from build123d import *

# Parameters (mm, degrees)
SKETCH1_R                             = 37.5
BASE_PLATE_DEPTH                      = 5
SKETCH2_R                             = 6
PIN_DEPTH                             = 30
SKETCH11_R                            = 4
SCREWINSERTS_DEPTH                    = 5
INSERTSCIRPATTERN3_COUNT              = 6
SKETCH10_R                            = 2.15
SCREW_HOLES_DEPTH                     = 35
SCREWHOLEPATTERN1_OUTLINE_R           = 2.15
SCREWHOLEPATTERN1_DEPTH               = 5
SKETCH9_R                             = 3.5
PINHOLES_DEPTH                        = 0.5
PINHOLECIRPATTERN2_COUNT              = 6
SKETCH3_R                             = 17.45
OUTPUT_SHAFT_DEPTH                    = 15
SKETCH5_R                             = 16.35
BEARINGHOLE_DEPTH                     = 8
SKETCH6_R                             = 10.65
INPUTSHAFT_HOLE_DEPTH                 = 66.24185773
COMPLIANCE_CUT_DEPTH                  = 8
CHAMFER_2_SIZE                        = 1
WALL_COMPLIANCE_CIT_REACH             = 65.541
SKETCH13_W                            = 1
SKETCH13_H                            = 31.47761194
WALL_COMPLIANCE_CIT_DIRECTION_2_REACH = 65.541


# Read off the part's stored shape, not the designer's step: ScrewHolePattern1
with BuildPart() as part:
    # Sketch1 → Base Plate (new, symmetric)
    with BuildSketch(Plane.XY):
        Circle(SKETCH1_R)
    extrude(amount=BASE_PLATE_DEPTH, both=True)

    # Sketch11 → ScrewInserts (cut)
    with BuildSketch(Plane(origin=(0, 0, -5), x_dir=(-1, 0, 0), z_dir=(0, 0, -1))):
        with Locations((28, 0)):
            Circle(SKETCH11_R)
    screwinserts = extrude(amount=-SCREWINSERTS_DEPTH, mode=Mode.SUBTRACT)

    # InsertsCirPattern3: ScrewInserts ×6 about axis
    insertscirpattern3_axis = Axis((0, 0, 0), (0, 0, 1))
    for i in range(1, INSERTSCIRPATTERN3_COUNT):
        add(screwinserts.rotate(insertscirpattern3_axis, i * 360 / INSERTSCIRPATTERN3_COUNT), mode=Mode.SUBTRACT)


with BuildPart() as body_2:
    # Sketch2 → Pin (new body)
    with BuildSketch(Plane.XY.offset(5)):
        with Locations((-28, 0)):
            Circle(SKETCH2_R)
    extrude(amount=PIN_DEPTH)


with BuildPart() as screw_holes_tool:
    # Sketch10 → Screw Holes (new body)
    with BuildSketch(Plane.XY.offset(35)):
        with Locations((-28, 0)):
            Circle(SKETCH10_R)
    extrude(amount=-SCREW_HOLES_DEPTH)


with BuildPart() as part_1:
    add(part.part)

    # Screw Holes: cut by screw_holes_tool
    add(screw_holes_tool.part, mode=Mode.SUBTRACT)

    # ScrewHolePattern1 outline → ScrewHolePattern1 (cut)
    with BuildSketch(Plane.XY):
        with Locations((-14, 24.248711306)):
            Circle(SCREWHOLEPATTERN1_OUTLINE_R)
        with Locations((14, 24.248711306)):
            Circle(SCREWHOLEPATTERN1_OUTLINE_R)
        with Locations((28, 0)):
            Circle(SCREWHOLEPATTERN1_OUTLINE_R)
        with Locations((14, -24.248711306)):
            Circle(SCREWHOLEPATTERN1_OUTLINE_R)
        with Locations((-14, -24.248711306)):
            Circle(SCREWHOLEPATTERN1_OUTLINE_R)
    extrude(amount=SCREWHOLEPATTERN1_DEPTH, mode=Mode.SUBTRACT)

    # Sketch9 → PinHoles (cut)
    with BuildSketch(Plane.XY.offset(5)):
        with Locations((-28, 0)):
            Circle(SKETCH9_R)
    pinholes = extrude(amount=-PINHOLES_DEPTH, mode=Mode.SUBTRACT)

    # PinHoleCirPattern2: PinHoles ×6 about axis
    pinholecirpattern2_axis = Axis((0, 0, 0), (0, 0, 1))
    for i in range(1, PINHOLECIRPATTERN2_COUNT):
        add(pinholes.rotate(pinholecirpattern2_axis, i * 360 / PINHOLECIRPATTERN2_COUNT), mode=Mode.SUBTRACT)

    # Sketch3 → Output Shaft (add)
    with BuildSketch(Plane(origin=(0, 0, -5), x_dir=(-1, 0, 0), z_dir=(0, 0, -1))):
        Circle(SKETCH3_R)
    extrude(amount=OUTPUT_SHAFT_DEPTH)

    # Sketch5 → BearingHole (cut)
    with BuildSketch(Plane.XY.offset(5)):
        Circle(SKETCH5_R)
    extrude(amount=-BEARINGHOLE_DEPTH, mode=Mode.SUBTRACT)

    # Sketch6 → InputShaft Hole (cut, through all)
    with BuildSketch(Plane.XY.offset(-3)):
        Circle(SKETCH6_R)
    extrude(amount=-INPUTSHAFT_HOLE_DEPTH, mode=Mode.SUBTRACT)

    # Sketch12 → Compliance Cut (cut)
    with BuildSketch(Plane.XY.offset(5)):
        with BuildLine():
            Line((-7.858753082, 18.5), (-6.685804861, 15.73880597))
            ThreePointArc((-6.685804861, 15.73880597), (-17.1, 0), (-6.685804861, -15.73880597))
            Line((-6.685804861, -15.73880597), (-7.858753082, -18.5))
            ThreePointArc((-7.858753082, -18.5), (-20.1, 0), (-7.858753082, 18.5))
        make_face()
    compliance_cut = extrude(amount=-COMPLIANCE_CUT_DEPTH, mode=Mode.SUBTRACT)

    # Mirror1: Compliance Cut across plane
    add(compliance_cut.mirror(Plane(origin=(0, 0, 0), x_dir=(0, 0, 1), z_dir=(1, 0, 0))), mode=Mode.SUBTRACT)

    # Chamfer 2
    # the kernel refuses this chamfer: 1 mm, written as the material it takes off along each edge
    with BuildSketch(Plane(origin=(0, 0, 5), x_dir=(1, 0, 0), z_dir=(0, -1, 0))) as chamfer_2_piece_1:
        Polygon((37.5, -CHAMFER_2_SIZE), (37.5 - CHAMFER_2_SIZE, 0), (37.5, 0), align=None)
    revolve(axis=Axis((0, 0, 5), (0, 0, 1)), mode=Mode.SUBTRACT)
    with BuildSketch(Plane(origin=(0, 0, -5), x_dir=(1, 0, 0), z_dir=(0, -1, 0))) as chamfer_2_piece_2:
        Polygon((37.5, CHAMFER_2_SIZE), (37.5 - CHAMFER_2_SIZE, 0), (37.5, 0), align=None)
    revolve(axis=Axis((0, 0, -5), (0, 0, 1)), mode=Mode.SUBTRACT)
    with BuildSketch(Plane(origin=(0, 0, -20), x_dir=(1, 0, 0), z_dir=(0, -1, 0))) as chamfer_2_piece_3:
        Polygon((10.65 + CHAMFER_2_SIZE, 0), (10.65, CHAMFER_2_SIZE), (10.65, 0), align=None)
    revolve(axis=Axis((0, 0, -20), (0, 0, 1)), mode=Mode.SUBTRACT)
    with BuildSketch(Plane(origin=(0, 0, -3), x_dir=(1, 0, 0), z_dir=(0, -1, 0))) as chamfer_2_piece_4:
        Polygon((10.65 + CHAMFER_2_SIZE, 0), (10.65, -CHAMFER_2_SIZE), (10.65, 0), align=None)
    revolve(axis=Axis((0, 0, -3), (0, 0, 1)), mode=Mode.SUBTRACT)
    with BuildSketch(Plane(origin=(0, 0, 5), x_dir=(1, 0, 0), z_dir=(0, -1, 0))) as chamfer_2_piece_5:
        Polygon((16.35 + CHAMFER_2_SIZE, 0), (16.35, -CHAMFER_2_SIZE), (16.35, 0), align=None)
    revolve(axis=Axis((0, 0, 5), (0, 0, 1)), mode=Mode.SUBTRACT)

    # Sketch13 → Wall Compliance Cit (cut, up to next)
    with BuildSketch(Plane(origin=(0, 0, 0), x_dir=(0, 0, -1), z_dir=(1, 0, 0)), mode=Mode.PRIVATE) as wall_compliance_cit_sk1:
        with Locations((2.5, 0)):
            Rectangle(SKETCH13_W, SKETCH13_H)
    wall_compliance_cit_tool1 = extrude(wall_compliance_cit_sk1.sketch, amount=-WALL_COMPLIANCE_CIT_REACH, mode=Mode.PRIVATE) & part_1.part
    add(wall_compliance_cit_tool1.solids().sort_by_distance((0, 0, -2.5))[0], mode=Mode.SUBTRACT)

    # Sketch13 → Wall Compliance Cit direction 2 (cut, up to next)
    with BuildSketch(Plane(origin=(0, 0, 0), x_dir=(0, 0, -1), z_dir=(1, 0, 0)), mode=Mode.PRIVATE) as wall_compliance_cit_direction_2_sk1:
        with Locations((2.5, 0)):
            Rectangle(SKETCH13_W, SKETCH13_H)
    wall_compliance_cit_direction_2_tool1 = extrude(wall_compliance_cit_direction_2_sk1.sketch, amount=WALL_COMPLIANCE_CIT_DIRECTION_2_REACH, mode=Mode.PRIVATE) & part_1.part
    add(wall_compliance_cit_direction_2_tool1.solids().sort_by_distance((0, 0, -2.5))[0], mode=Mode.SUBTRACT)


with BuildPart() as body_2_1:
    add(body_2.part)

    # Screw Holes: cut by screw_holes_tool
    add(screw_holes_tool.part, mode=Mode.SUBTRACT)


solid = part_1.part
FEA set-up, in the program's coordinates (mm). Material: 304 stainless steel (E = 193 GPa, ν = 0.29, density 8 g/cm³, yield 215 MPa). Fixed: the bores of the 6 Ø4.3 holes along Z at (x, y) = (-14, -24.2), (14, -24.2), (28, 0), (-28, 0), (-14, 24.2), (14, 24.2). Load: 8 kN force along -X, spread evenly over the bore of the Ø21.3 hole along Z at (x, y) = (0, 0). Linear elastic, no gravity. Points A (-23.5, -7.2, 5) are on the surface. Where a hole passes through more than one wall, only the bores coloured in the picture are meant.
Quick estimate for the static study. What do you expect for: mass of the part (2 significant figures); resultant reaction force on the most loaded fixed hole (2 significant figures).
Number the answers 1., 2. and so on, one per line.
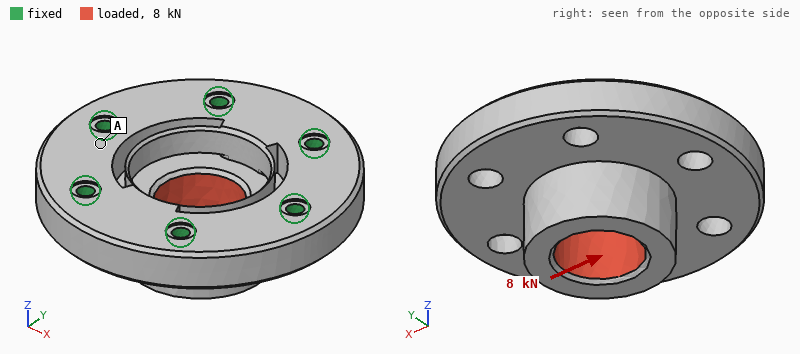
1. 330 g
2. 2.0 kN
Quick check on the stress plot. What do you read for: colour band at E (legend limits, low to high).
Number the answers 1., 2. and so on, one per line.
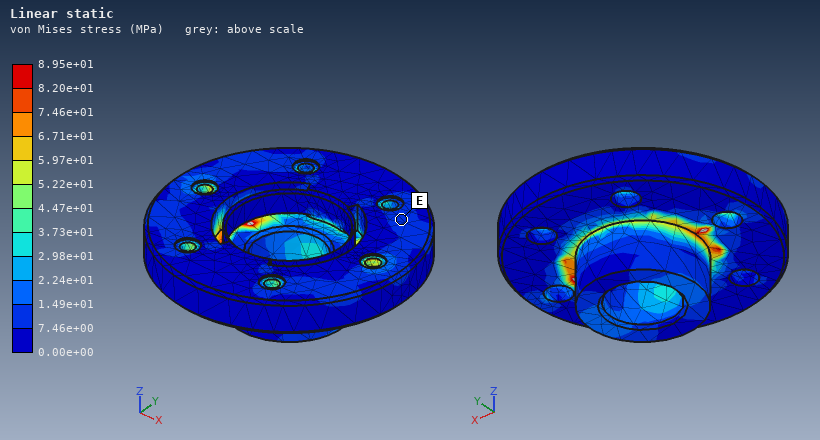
1. 7.46e+00 to 1.49e+01 MPa
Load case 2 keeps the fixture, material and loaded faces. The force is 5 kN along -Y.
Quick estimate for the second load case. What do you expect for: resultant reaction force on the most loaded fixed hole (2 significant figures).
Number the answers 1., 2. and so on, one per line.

1. 1.2 kN
